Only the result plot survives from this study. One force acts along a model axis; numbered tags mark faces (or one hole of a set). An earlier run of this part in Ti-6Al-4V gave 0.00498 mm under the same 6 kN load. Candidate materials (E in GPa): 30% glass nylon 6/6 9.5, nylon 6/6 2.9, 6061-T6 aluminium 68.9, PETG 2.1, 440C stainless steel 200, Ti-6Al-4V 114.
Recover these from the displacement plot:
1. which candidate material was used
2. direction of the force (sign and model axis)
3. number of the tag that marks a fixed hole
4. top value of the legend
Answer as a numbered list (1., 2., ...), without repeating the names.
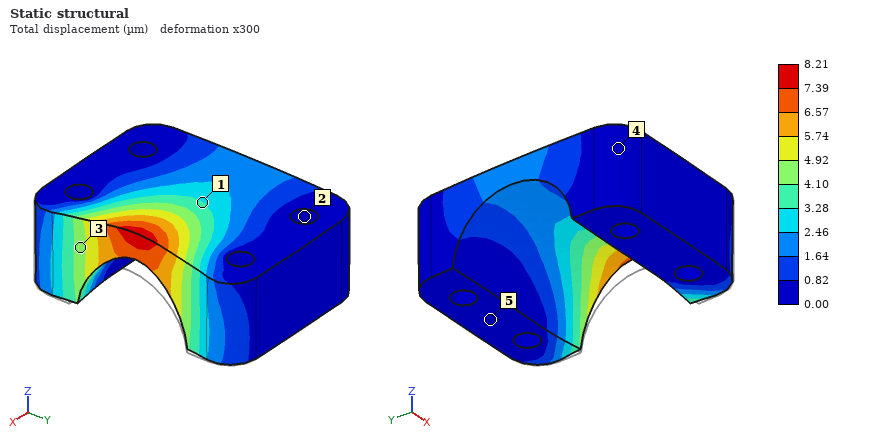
1. 6061-T6 aluminium
2. -X
3. 2
4. 8.21 µm
